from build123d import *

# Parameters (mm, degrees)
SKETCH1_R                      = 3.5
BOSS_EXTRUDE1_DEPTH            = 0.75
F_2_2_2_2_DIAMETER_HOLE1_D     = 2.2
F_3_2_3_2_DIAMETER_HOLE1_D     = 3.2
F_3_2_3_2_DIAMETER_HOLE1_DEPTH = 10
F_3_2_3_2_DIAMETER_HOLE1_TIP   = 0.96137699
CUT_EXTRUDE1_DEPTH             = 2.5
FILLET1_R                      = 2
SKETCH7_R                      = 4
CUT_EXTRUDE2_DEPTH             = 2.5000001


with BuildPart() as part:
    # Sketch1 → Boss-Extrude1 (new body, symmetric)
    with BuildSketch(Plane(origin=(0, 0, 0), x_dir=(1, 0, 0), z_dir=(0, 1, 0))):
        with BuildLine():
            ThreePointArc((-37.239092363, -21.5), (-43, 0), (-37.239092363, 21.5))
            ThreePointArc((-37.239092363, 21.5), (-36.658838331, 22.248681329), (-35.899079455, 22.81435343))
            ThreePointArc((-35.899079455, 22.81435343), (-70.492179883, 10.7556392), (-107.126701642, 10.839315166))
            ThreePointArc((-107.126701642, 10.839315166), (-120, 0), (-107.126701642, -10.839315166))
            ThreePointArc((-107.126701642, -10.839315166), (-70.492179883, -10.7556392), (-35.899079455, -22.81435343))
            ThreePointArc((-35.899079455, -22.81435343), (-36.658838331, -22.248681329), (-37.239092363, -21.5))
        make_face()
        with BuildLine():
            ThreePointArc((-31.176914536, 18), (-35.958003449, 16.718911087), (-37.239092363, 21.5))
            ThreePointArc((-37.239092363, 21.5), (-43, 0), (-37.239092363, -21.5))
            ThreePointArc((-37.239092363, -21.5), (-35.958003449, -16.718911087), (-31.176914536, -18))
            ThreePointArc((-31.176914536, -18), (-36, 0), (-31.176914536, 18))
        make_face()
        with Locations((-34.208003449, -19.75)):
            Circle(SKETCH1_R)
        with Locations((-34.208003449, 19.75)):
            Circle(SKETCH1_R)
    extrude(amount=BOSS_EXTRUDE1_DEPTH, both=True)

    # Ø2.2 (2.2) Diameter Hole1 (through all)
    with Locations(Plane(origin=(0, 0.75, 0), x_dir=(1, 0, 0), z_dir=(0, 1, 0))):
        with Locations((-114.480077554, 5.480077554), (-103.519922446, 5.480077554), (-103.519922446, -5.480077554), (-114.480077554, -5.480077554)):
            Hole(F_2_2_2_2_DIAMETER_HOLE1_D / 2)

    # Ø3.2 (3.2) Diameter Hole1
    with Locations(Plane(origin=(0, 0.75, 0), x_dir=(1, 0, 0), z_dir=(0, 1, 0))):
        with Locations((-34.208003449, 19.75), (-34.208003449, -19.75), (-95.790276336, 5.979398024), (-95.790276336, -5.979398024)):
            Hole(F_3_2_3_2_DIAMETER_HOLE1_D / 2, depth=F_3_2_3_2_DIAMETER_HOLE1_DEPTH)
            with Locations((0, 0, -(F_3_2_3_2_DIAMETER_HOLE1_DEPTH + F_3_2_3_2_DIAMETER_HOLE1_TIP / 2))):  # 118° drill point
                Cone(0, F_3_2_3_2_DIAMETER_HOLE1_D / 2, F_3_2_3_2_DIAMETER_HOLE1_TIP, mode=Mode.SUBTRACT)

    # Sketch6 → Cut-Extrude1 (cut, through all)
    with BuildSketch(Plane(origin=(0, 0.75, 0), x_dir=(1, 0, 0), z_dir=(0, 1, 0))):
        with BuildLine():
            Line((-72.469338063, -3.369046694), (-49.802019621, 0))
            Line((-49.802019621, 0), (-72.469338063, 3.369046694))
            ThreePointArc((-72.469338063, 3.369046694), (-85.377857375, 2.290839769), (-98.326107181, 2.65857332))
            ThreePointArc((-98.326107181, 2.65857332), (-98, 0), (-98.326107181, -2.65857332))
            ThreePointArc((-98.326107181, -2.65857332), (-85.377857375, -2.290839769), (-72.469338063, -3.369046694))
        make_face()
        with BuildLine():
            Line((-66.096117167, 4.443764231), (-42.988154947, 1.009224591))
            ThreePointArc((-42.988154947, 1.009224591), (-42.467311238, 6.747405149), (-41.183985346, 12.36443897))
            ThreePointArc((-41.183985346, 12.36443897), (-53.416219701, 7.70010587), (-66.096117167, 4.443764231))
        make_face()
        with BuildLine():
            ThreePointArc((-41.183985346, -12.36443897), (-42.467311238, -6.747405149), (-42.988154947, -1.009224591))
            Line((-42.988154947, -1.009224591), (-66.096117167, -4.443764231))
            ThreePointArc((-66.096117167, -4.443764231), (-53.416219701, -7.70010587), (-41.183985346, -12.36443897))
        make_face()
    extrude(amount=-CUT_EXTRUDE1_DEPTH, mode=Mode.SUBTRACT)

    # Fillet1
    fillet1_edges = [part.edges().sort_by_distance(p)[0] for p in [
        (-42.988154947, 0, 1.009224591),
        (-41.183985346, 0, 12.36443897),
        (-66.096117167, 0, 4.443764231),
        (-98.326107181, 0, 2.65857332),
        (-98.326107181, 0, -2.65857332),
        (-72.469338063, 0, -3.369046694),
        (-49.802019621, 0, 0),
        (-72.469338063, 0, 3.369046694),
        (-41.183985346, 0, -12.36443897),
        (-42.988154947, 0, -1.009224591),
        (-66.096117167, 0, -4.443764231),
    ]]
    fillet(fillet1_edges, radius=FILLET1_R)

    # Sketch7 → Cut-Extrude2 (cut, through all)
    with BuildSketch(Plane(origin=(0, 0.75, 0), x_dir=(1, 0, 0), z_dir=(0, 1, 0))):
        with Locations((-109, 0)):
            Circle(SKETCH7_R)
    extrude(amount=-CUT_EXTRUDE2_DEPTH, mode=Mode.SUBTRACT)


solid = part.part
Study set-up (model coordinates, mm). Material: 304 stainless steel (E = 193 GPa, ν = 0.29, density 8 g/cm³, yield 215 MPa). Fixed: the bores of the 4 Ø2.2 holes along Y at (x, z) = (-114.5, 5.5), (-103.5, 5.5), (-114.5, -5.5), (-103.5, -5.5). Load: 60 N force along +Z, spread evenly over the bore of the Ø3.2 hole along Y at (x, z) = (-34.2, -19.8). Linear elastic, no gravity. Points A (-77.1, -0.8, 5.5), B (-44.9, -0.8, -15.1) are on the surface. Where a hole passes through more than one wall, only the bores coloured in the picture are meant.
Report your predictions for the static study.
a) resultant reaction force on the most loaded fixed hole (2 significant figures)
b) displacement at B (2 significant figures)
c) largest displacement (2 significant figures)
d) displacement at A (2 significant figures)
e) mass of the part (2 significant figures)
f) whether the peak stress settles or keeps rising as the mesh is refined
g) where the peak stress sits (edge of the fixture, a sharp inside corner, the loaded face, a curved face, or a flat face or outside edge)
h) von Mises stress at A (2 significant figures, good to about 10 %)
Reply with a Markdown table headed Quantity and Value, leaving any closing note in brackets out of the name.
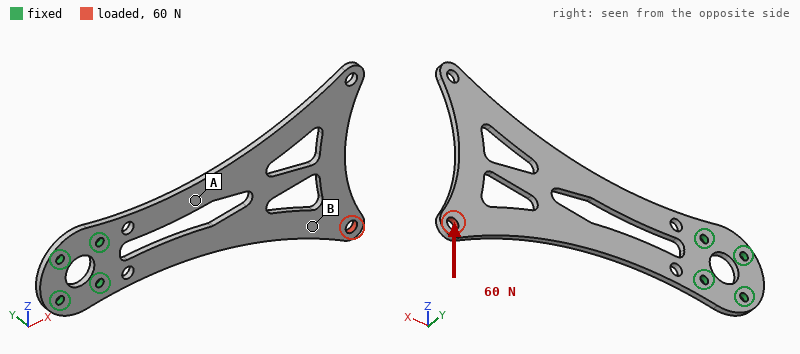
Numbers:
| Quantity | Value |
|---|---|
| resultant reaction force on the most loaded fixed hole | 250 N |
| displacement at B | 66 µm |
| largest displacement | 85 µm |
| displacement at A | 23 µm |
| mass of the part | 20 g |
| whether the peak stress settles or keeps rising as the mesh is refined | keeps rising |
| where the peak stress sits | a sharp inside corner |
| von Mises stress at A | 22 MPa |
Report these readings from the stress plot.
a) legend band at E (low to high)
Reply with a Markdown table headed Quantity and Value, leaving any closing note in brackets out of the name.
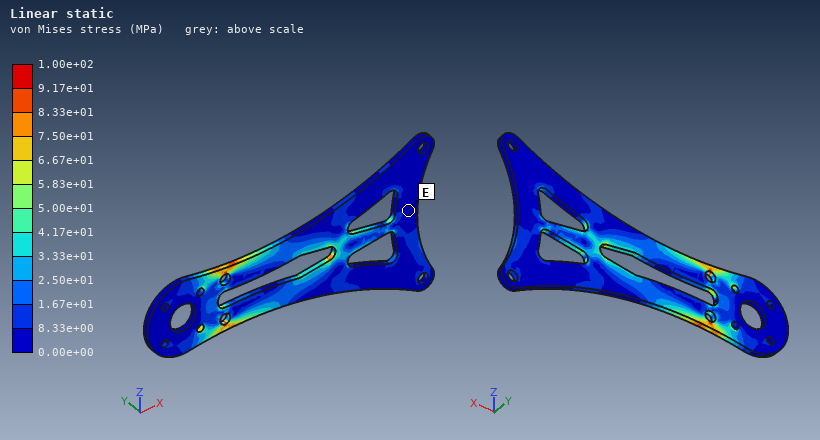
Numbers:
| Quantity | Value |
|---|---|
| legend band at E | 0.00e+00 to 8.33e+00 MPa |
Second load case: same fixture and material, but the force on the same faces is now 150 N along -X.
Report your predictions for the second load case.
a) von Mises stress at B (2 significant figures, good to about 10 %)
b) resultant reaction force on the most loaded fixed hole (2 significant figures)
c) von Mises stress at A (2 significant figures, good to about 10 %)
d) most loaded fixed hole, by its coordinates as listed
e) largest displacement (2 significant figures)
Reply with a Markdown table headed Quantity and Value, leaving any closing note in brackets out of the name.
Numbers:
| Quantity | Value |
|---|---|
| von Mises stress at B | 16 MPa |
| resultant reaction force on the most loaded fixed hole | 260 N |
| von Mises stress at A | 11 MPa |
| most loaded fixed hole, by its coordinates as listed | (-103.5, -5.5) |
| largest displacement | 65 µm |
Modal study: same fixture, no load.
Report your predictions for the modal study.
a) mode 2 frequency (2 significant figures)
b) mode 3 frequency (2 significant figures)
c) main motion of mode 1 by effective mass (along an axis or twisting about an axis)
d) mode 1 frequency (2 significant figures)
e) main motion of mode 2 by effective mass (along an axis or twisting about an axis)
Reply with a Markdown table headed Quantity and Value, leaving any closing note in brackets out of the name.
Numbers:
| Quantity | Value |
|---|---|
| mode 2 frequency | 640 Hz |
| mode 3 frequency | 1300 Hz |
| main motion of mode 1 by effective mass | along Y |
| mode 1 frequency | 170 Hz |
| main motion of mode 2 by effective mass | twisting about X |
